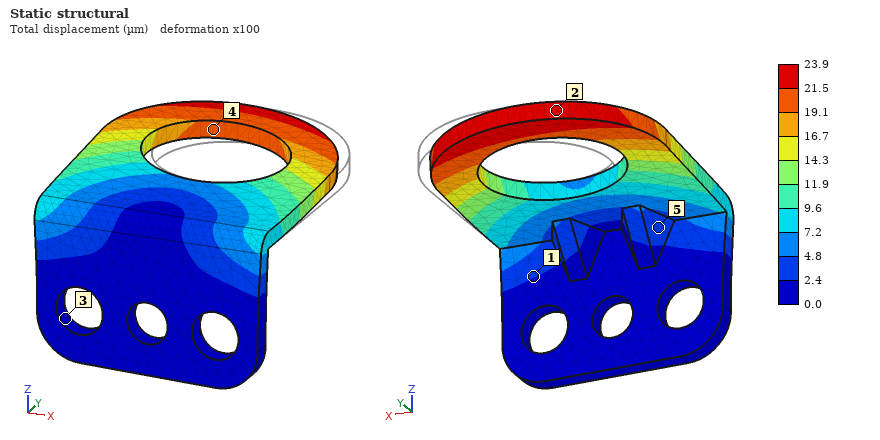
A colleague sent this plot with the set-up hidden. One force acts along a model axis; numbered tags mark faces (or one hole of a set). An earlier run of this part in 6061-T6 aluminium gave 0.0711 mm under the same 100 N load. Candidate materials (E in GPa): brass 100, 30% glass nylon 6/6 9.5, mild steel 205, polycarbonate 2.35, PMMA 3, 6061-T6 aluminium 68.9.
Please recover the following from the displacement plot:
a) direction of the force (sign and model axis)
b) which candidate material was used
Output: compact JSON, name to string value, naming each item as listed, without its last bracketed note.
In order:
{"direction of the force": "-X", "which candidate material was used": "mild steel"}
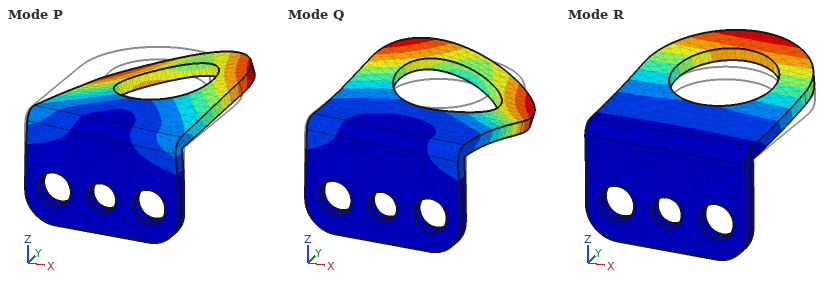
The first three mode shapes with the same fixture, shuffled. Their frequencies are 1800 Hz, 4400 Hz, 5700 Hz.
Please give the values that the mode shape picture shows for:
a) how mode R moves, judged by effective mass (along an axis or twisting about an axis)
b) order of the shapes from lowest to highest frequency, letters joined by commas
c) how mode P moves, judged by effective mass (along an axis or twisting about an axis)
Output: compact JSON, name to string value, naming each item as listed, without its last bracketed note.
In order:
{"how mode R moves, judged by effective mass": "along Z", "order of the shapes from lowest to highest frequency, letters joined by commas": "R, P, Q", "how mode P moves, judged by effective mass": "along X"}
